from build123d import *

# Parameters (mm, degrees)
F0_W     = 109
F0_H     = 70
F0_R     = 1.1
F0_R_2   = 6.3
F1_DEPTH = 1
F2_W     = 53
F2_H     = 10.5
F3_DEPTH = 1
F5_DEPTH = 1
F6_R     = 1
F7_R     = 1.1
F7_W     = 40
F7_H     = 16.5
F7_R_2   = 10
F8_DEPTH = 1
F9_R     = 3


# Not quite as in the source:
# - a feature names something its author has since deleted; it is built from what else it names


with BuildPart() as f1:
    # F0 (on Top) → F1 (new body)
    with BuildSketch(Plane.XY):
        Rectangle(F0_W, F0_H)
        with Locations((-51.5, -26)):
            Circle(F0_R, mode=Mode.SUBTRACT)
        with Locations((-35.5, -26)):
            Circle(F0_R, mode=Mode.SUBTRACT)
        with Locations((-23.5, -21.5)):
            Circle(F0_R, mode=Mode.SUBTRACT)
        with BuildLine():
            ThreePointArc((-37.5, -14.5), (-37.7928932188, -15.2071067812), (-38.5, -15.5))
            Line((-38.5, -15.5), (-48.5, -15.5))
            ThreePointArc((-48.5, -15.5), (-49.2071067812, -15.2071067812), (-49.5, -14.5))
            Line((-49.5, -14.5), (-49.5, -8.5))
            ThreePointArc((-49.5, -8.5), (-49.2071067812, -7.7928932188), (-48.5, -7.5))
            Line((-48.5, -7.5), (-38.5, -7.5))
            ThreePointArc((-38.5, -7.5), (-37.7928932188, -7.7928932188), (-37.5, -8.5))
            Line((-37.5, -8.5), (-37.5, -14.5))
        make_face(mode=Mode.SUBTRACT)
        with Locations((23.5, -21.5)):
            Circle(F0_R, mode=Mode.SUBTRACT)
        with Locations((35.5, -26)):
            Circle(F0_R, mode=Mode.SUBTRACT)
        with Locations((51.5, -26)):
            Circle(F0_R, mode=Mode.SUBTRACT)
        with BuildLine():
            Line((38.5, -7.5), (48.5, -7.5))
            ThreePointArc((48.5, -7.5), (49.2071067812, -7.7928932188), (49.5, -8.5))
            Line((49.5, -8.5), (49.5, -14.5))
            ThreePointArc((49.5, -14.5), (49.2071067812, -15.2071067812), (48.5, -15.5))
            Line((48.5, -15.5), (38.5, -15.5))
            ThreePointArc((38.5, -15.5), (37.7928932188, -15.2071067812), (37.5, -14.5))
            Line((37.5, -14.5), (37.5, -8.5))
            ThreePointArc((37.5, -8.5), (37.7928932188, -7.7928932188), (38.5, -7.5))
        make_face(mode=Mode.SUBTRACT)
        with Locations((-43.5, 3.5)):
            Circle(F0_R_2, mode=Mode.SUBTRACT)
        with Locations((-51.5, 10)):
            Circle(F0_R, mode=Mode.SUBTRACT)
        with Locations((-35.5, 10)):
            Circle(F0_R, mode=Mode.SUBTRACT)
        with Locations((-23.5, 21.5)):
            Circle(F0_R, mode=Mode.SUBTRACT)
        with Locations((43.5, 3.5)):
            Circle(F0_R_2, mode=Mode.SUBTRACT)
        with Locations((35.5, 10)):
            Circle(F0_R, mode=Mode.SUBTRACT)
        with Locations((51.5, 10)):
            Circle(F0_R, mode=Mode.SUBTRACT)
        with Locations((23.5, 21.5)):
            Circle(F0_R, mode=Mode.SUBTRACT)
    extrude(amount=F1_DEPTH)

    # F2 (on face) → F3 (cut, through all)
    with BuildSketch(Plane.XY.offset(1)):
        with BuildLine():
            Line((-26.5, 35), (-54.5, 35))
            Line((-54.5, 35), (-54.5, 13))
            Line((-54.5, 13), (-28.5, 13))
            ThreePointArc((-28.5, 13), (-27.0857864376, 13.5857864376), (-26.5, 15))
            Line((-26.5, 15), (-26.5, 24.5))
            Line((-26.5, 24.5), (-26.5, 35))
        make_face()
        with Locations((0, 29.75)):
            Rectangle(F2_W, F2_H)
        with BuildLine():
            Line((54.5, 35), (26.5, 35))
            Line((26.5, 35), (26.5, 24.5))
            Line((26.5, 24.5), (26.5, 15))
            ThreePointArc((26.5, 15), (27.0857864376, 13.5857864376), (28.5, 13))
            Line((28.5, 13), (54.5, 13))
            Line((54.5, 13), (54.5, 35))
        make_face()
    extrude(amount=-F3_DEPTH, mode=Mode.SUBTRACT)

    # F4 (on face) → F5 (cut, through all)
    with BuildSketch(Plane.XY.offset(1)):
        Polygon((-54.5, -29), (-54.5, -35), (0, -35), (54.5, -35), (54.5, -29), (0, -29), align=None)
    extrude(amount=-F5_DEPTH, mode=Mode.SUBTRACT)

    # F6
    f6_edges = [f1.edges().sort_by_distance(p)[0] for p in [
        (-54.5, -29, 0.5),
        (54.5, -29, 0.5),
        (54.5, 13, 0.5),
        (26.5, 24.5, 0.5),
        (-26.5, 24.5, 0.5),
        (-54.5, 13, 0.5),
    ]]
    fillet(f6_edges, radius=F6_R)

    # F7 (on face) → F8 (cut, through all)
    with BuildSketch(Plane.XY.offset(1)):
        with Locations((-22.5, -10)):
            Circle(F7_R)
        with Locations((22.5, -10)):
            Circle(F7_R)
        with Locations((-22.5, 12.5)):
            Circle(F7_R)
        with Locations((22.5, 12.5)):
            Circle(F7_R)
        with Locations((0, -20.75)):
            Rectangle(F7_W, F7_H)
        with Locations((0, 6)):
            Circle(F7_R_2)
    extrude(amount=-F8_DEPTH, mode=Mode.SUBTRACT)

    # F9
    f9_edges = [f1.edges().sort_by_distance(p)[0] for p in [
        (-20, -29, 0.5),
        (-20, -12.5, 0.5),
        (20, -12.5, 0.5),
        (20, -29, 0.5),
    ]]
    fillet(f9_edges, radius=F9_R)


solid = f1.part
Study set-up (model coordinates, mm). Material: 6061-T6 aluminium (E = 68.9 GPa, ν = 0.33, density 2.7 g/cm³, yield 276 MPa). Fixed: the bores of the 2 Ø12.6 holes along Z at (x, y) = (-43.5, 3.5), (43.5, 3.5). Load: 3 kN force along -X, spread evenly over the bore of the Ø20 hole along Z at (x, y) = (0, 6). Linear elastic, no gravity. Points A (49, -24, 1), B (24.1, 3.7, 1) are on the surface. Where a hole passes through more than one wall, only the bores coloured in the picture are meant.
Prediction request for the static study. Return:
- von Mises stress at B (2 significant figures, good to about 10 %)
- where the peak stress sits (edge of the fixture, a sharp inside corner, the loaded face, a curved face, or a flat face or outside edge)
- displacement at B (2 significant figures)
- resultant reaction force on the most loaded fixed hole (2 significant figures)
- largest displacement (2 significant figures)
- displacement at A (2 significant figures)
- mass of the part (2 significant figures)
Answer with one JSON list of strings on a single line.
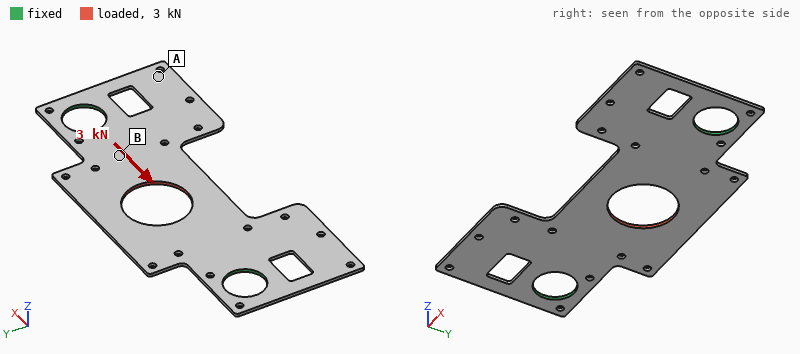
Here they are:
["65 MPa", "a curved face", "15 µm", "1.5 kN", "46 µm", "15 µm", "10 g"]
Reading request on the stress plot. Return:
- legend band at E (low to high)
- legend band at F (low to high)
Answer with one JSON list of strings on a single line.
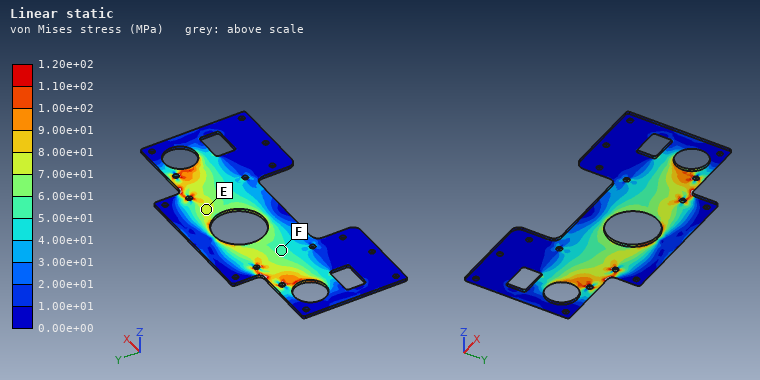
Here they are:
["7.00e+01 to 8.00e+01 MPa", "5.00e+01 to 6.00e+01 MPa"]
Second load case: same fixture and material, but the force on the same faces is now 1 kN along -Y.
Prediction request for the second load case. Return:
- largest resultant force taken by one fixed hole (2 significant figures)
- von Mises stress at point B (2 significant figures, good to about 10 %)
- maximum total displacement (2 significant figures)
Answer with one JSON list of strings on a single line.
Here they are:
["500 N", "36 MPa", "50 µm"]
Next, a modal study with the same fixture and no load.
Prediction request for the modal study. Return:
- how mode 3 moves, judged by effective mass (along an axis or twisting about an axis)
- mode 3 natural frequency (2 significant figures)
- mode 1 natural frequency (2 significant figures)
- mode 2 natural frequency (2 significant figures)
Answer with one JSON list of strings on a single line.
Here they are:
["twisting about Y", "910 Hz", "760 Hz", "780 Hz"]
